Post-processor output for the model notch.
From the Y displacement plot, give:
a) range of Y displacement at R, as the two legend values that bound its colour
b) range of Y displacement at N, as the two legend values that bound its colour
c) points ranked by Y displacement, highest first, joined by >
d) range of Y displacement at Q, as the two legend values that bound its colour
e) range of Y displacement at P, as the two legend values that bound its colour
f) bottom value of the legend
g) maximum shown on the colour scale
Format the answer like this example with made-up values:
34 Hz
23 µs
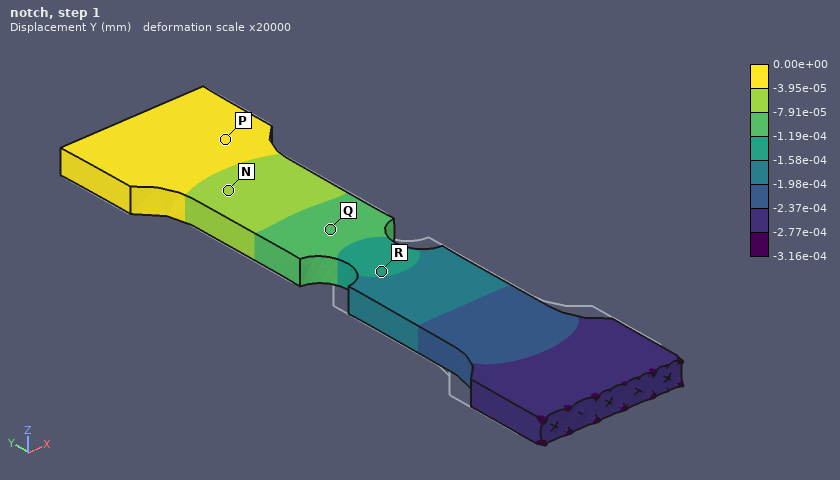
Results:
-1.58e-04 to -1.19e-04 mm
-7.91e-05 to -3.95e-05 mm
P > N > Q > R
-1.19e-04 to -7.91e-05 mm
-3.95e-05 to 0.00e+00 mm
-3.16e-04 mm
0.00e+00 mm
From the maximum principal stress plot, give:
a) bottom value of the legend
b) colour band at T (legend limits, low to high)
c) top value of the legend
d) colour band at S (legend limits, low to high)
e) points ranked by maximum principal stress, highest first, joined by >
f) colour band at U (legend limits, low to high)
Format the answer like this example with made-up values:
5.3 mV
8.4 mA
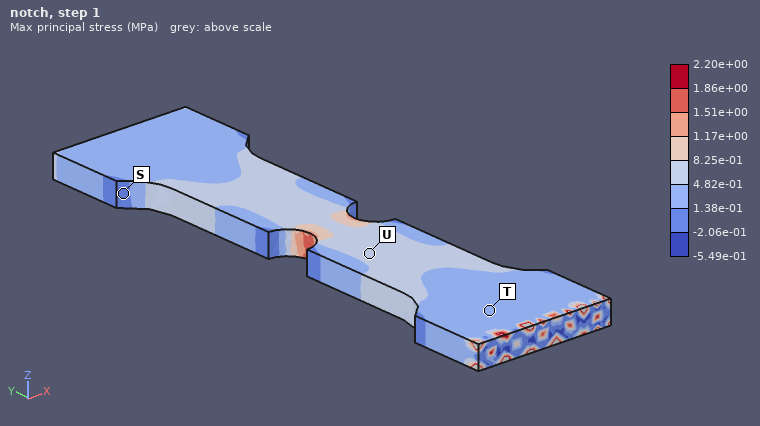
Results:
-5.49e-01 MPa
1.38e-01 to 4.82e-01 MPa
2.20e+00 MPa
-2.06e-01 to 1.38e-01 MPa
U > T > S
4.82e-01 to 8.25e-01 MPa
